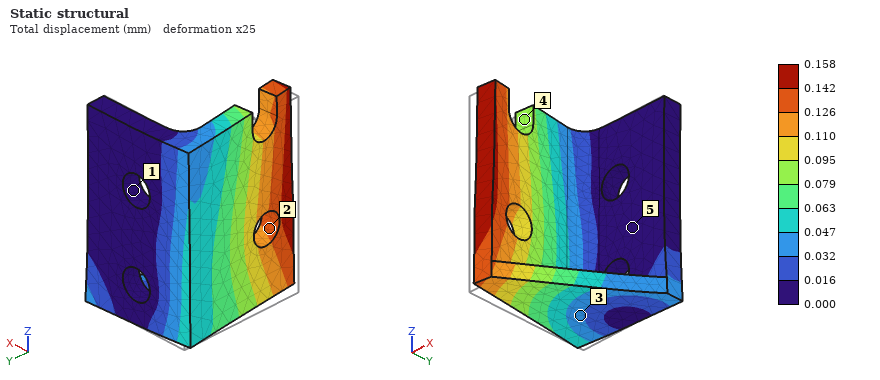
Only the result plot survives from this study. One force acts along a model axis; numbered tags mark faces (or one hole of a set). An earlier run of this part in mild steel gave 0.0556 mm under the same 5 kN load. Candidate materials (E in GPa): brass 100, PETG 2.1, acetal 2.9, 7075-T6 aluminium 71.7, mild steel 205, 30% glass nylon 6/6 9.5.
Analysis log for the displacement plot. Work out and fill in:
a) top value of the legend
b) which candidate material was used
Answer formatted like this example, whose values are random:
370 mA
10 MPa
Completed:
0.158 mm
7075-T6 aluminium
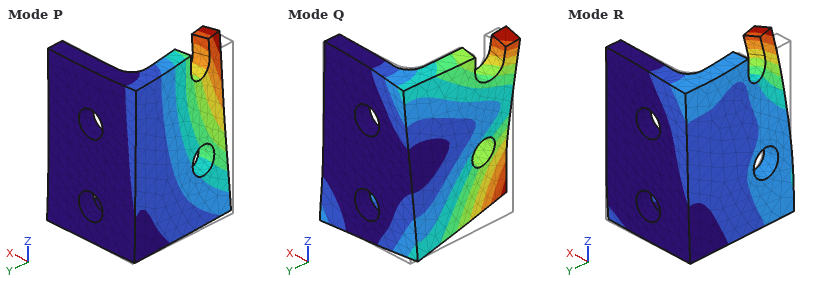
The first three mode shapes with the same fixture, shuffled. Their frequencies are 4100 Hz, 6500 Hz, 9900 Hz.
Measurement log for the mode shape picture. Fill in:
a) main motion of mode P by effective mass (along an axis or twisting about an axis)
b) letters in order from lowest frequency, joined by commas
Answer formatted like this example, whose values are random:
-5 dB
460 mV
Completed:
along X
P, Q, R
